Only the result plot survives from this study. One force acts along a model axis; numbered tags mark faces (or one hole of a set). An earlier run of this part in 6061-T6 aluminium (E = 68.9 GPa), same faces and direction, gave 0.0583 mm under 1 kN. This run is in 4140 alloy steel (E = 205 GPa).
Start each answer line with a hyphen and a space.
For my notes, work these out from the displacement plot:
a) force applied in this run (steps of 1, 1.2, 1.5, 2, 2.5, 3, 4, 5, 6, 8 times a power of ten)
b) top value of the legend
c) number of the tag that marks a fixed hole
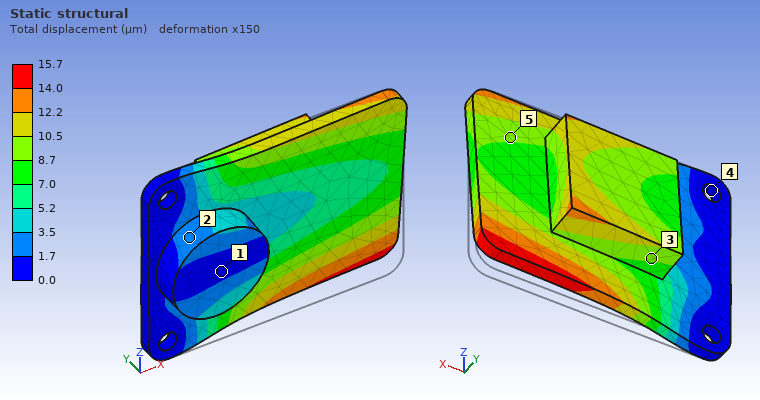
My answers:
- 800 N
- 15.7 µm
- 4
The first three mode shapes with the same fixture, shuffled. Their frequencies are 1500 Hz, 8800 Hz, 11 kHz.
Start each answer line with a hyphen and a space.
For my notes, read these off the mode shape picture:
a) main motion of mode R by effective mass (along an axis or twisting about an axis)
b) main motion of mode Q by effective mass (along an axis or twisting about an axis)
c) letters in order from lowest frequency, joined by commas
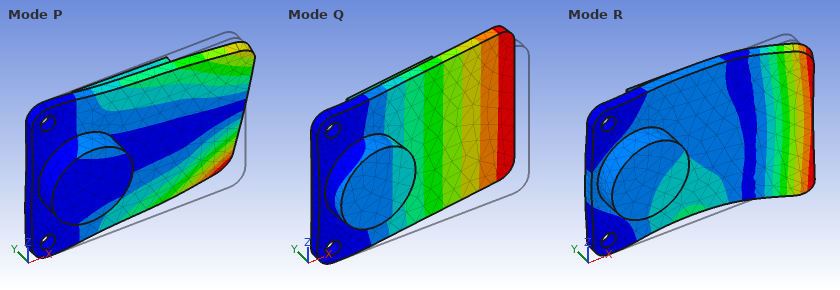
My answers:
- along Y
- along Y
- Q, P, R
